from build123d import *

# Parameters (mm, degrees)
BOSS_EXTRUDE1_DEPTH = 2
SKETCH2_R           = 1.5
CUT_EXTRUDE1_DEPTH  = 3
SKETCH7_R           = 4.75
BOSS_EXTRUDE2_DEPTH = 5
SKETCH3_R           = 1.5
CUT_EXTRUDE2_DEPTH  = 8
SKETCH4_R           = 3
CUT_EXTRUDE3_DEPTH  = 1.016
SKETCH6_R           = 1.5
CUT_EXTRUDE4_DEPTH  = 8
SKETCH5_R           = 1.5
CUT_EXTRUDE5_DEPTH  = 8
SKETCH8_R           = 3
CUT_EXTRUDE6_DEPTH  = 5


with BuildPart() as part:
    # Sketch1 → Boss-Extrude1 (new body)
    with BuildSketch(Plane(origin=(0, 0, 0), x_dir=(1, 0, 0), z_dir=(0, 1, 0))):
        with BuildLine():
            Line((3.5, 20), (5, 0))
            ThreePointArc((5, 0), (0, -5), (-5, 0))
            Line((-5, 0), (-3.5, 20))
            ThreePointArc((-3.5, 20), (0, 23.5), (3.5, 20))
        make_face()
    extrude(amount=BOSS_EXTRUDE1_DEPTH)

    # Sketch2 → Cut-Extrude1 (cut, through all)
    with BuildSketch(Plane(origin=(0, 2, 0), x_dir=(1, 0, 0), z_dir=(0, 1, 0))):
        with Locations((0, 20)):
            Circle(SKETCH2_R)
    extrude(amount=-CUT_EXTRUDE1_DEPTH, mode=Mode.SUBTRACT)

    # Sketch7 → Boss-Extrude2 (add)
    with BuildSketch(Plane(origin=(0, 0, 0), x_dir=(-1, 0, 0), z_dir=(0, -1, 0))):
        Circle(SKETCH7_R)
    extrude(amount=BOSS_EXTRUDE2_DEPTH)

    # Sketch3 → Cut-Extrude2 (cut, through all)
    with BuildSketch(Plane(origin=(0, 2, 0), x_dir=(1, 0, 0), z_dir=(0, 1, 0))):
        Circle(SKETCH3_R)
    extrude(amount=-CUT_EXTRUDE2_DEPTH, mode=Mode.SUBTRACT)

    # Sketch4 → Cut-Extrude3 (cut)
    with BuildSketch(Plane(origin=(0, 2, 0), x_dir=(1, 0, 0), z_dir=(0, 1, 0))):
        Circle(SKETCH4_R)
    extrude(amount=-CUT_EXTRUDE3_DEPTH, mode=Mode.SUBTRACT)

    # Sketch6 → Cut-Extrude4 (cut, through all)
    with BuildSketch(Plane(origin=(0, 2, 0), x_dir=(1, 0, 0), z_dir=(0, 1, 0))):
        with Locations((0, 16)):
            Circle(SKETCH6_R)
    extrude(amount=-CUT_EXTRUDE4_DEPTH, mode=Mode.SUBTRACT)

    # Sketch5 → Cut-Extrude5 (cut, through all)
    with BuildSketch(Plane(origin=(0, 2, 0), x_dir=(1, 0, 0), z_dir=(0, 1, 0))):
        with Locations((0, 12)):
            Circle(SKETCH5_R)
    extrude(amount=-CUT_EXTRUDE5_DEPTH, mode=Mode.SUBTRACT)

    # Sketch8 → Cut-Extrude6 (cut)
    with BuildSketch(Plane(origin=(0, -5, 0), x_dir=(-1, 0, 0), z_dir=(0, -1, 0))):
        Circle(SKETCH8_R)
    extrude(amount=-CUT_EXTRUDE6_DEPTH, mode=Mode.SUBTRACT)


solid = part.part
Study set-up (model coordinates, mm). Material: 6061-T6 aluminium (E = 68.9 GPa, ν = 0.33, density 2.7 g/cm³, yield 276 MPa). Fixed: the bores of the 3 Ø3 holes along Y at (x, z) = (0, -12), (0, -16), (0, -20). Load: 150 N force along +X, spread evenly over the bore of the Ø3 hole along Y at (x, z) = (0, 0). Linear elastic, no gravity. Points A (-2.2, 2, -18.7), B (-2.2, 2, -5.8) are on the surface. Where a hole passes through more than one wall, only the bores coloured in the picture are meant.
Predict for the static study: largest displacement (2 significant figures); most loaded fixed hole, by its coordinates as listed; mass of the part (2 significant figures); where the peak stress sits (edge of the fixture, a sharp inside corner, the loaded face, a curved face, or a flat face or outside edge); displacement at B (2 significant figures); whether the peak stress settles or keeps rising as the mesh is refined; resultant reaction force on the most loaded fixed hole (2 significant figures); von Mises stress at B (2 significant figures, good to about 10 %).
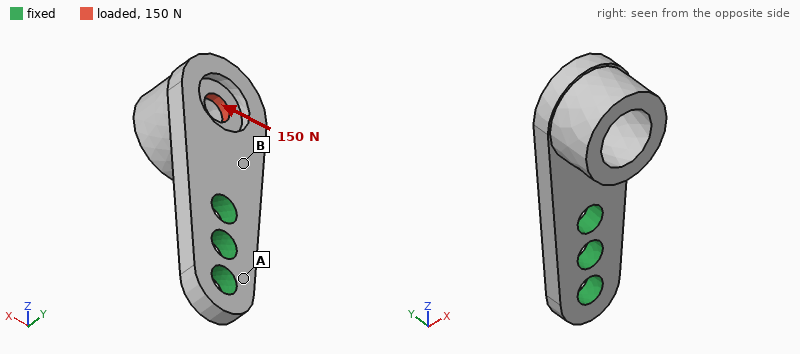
35 µm
(0, -12)
1.6 g
edge of the fixture
9.2 µm
keeps rising
280 N
15 MPa
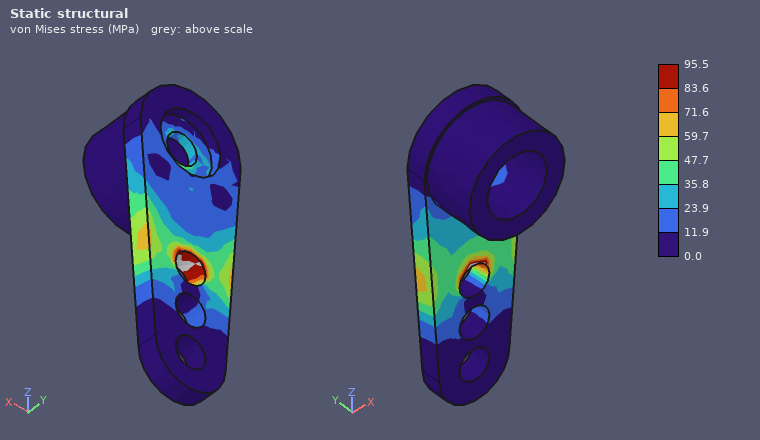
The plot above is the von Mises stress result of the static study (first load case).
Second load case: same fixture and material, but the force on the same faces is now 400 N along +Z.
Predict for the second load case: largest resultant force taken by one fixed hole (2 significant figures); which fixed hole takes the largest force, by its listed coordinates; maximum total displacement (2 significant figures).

340 N
(0, -12)
49 µm
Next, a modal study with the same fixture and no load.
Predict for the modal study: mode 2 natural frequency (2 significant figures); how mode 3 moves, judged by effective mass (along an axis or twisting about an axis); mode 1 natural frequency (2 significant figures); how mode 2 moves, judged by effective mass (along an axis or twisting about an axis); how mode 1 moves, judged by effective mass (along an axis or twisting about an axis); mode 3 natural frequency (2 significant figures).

10000 Hz
along X
4400 Hz
along X
along Y
16 kHz
